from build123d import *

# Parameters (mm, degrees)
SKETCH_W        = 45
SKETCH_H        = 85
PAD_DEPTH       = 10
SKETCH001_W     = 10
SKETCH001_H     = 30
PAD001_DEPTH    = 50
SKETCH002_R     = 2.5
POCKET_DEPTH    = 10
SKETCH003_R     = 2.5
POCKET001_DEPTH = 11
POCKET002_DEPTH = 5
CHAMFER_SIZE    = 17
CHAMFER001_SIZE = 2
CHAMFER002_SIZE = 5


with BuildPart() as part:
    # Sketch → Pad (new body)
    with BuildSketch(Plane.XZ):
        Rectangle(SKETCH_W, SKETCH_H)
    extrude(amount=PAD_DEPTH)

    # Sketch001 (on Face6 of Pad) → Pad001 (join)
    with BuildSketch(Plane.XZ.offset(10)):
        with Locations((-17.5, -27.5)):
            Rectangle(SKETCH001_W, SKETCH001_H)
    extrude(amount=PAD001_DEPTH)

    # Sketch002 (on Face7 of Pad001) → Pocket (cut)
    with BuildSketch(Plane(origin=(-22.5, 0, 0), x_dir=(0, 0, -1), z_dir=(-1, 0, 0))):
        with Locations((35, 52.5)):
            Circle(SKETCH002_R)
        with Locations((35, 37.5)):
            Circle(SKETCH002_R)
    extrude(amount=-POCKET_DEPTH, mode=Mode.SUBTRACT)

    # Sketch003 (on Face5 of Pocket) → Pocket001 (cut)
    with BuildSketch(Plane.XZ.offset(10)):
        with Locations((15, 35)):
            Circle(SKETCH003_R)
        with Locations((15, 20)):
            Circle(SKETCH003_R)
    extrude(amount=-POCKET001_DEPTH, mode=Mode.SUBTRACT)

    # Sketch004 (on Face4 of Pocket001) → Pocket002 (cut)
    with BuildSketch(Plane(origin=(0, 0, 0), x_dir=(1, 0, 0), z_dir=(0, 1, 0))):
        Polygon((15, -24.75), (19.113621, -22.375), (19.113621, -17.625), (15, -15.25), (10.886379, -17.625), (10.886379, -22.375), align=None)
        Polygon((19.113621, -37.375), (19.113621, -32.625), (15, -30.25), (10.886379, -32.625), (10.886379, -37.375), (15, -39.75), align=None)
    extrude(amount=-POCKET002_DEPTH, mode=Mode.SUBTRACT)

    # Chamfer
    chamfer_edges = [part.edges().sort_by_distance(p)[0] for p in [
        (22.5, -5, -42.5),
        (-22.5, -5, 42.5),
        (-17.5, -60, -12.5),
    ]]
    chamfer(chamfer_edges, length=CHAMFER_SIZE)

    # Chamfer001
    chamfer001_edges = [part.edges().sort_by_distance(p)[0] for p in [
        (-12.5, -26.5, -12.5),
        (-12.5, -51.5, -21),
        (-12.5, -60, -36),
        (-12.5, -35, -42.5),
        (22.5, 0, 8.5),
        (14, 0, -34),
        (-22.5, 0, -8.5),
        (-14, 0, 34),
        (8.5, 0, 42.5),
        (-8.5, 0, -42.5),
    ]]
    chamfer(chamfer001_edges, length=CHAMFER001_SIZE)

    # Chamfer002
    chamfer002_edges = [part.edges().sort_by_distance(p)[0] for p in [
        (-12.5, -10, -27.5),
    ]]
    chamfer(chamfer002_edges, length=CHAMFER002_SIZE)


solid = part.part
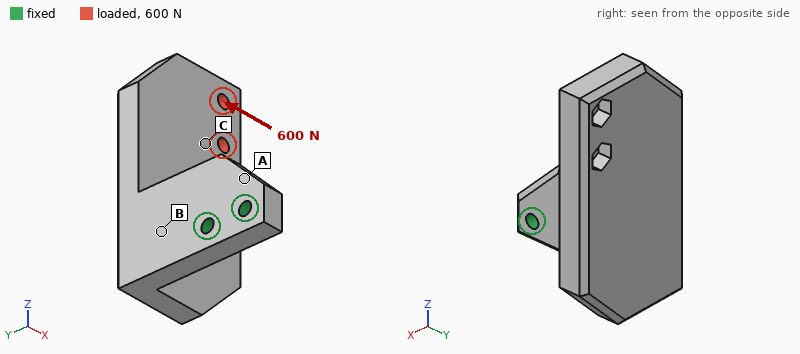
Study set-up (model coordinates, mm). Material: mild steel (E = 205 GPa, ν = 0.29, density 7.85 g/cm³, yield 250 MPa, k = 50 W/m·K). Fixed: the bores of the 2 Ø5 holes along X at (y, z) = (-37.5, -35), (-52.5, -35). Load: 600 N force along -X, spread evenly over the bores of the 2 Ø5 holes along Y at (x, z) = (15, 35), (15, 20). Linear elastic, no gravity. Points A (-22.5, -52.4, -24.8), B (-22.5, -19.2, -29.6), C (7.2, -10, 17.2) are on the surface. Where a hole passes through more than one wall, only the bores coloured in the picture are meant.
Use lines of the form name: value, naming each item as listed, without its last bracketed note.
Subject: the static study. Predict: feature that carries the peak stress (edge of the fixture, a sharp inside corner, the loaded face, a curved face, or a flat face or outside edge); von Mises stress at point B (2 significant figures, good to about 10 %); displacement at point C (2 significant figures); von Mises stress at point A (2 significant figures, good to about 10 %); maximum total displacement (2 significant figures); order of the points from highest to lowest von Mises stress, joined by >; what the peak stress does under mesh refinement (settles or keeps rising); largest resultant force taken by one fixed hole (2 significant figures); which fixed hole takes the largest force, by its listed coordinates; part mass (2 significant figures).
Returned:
feature that carries the peak stress: edge of the fixture
von Mises stress at point B: 58 MPa
displacement at point C: 0.11 mm
von Mises stress at point A: 33 MPa
maximum total displacement: 0.17 mm
order of the points from highest to lowest von Mises stress, joined by >: B > A > C
what the peak stress does under mesh refinement: keeps rising
largest resultant force taken by one fixed hole: 1.0 kN
which fixed hole takes the largest force, by its listed coordinates: (-37.5, -35)
part mass: 370 g
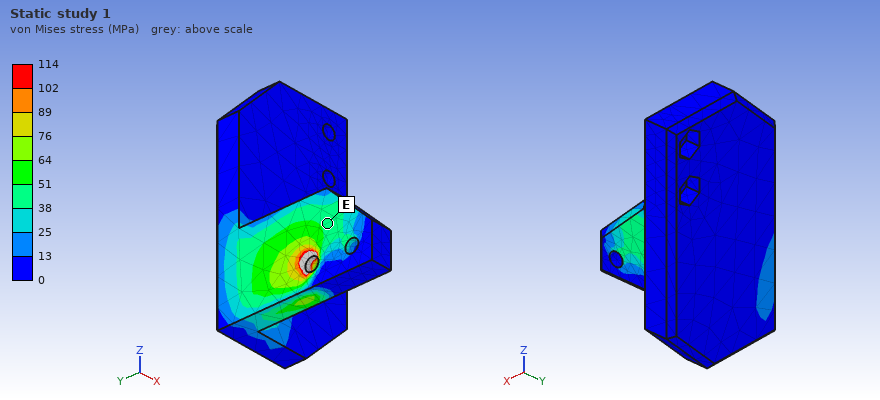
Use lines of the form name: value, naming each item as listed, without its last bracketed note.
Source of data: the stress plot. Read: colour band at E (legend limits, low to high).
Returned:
colour band at E: 38 to 51 MPa
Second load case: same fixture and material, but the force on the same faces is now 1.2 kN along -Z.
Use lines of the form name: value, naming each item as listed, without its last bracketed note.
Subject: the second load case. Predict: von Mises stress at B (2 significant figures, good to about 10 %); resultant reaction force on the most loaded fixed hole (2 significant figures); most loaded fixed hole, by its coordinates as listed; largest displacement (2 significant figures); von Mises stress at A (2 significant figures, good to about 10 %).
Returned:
von Mises stress at B: 55 MPa
resultant reaction force on the most loaded fixed hole: 2.9 kN
most loaded fixed hole, by its coordinates as listed: (-37.5, -35)
largest displacement: 0.17 mm
von Mises stress at A: 48 MPa
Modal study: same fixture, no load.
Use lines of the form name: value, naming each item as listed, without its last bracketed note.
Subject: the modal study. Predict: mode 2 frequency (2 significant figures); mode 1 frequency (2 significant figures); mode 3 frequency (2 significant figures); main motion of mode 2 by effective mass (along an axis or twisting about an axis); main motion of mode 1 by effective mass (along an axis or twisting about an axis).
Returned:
mode 2 frequency: 1300 Hz
mode 1 frequency: 870 Hz
mode 3 frequency: 2300 Hz
main motion of mode 2 by effective mass: along Y
main motion of mode 1 by effective mass: along X
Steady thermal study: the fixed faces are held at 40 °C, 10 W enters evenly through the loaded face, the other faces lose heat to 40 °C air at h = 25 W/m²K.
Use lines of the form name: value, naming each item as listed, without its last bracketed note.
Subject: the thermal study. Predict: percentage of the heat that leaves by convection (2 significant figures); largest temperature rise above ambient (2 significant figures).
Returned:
percentage of the heat that leaves by convection: 51 %
largest temperature rise above ambient: 38 K
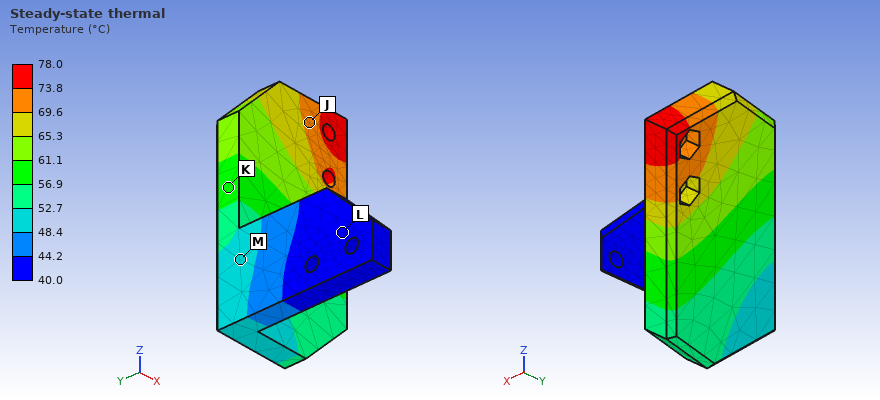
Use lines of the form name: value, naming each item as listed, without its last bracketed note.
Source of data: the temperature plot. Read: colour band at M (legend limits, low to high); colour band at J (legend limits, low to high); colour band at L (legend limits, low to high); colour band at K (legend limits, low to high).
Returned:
colour band at M: 48.4 to 52.7 °C
colour band at J: 69.6 to 73.8 °C
colour band at L: 40.0 to 44.2 °C
colour band at K: 56.9 to 61.1 °C
